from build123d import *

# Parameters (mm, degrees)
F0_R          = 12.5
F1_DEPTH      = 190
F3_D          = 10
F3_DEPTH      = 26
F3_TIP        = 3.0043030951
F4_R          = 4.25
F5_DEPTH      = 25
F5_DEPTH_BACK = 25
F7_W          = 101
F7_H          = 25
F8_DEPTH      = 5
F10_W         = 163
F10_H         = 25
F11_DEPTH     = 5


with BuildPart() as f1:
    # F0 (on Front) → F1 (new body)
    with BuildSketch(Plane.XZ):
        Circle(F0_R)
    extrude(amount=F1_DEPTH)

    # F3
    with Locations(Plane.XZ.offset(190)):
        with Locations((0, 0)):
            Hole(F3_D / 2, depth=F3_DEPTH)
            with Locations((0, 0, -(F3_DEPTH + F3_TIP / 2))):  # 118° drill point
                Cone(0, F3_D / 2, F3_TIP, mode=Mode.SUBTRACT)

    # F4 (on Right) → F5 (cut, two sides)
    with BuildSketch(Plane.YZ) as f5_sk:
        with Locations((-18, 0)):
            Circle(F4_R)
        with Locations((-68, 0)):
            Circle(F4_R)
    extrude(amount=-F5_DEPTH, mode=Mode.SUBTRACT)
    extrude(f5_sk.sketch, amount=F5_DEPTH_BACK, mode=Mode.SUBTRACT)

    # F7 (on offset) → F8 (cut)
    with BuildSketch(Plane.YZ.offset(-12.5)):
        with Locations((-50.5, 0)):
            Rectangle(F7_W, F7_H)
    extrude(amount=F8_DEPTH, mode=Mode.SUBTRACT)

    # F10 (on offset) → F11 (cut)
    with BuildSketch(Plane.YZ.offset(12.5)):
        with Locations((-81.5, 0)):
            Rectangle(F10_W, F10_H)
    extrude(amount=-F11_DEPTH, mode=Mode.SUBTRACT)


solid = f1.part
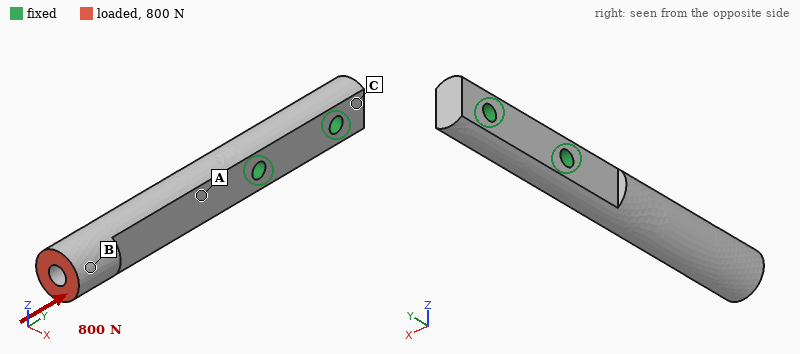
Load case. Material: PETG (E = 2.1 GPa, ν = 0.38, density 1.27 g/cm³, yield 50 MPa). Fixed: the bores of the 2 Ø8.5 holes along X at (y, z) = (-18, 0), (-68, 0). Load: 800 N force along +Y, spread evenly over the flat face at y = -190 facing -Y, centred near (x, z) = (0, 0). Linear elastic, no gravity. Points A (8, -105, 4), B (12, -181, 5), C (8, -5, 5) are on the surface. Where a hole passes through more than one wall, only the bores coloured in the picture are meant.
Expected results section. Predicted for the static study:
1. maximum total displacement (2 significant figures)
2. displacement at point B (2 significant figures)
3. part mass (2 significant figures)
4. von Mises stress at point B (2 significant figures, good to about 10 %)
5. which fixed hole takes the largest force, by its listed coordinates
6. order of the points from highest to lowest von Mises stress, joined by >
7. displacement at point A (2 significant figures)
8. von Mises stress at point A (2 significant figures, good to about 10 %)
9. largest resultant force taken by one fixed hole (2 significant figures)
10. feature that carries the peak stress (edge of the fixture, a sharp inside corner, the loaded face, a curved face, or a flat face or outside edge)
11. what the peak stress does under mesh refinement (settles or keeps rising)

0.25 mm
0.22 mm
90 g
1.9 MPa
(-68, 0)
A > B > C
0.041 mm
2.6 MPa
760 N
edge of the fixture
keeps rising
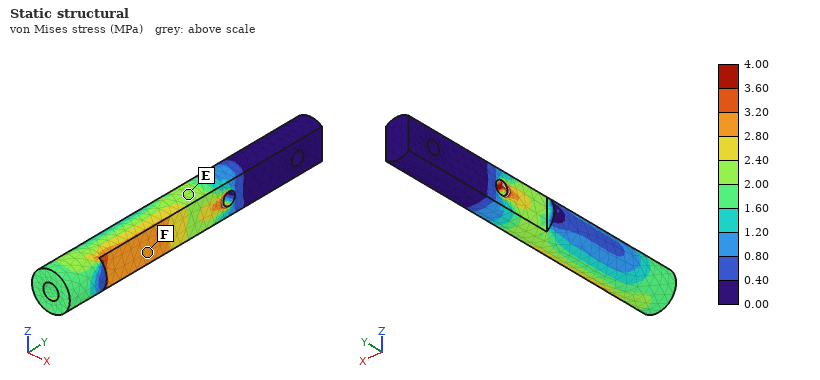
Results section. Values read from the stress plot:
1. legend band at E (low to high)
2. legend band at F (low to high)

2.00 to 2.40 MPa
2.80 to 3.20 MPa
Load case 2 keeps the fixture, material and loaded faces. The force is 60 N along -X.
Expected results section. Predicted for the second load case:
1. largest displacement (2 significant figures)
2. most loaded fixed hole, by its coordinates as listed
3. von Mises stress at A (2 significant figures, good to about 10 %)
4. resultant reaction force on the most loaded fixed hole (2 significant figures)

2.3 mm
(-68, 0)
5.1 MPa
72 N
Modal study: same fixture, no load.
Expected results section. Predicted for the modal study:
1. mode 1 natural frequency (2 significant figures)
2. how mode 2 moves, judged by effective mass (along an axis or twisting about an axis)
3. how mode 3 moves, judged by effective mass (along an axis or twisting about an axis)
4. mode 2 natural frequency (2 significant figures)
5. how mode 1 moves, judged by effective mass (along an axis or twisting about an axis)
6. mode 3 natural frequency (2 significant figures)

200 Hz
along Z
twisting about Y
270 Hz
along X
1300 Hz
